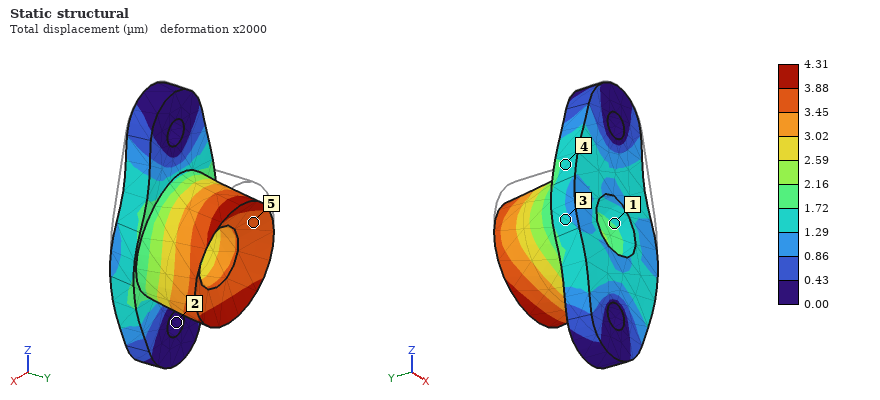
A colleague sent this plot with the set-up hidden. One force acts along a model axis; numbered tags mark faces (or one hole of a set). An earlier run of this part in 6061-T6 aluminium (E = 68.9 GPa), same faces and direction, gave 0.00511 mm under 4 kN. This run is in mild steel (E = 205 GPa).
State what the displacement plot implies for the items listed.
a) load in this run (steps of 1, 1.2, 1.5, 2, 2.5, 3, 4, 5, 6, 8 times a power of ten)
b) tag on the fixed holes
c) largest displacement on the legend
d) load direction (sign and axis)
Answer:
10 kN
2
4.31 µm
-Z
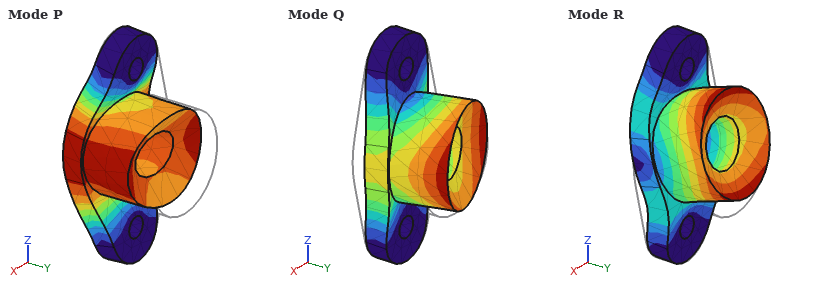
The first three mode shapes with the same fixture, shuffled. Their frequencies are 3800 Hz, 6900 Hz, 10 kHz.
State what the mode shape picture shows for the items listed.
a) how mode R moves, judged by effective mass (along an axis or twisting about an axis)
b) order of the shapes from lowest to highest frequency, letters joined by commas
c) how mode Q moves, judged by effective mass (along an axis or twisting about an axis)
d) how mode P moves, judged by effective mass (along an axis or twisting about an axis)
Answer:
along Z
Q, P, R
along X
along Y
